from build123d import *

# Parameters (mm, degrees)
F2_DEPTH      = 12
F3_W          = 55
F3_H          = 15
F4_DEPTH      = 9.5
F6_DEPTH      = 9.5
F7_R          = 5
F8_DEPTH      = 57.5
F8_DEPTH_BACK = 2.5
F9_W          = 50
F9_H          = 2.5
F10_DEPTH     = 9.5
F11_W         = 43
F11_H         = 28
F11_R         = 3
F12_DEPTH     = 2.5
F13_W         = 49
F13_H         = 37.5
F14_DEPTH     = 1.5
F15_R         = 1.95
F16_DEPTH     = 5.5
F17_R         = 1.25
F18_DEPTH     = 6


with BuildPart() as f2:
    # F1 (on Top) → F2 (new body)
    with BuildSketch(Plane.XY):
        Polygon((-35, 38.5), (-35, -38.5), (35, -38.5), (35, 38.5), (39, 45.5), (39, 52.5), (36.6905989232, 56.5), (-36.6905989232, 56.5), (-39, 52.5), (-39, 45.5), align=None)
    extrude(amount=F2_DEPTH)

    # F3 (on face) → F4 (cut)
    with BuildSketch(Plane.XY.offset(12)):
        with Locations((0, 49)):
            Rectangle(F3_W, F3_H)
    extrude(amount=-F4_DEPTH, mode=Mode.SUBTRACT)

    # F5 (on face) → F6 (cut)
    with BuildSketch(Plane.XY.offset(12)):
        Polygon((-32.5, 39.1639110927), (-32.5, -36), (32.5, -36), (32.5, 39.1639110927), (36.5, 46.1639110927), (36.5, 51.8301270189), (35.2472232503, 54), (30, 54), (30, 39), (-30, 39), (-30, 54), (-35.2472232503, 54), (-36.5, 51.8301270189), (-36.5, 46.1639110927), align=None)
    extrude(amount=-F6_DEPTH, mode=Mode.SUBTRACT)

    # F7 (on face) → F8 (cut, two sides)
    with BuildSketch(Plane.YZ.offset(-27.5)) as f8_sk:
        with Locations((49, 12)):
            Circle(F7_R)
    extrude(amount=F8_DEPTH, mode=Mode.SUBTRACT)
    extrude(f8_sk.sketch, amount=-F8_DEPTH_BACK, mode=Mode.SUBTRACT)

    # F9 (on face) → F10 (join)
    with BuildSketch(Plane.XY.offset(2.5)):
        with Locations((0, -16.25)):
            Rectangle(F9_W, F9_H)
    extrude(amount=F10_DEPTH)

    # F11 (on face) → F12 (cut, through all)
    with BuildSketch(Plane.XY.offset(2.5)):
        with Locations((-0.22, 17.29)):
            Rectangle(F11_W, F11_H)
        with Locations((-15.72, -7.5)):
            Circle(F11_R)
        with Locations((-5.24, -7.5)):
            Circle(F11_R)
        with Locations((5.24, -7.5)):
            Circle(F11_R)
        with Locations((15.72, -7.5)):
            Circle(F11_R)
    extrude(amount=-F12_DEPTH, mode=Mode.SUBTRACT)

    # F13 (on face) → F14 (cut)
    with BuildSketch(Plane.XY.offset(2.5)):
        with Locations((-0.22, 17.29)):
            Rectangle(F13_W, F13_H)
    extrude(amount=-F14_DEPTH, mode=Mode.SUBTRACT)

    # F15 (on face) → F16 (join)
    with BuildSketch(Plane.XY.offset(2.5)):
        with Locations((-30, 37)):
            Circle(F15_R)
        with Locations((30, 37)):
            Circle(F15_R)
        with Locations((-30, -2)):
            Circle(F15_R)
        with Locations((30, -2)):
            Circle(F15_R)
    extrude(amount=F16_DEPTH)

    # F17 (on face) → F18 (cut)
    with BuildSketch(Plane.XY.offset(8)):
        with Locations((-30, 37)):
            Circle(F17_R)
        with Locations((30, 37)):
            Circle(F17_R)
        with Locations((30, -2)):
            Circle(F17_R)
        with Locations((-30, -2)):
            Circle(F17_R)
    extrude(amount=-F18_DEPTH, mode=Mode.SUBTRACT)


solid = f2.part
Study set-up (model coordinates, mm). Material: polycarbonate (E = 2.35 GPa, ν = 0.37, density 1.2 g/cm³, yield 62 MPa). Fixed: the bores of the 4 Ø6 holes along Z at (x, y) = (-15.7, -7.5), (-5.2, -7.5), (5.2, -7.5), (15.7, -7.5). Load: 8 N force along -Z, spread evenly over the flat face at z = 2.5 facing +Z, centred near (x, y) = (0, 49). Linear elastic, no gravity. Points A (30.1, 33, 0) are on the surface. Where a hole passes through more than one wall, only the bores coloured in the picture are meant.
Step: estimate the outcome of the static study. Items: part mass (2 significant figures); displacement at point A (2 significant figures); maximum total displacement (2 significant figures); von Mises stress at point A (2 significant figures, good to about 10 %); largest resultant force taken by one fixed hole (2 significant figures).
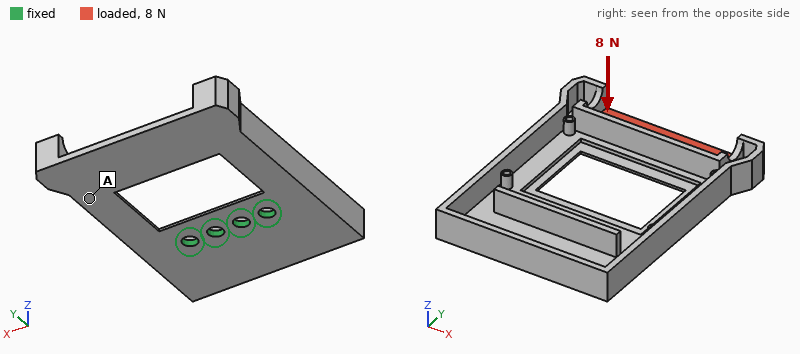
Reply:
27 g
0.82 mm
1.4 mm
1.0 MPa
10 N
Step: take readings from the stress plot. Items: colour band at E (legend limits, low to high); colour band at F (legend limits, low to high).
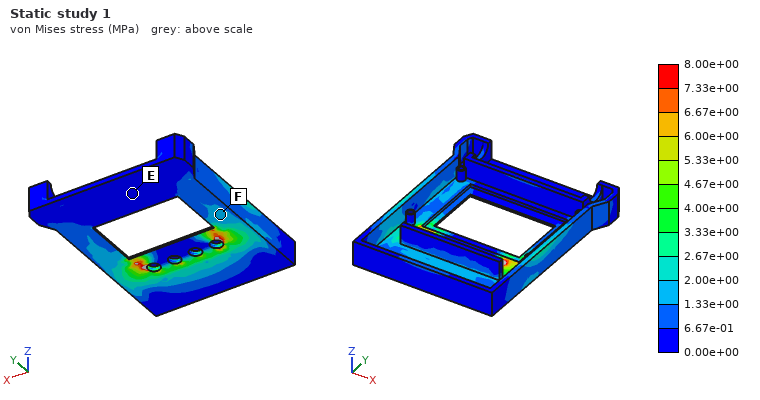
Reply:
0.00e+00 to 6.67e-01 MPa
1.33e+00 to 2.00e+00 MPa
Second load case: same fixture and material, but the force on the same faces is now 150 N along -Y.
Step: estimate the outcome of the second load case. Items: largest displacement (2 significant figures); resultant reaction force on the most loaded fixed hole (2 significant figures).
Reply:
0.57 mm
79 N
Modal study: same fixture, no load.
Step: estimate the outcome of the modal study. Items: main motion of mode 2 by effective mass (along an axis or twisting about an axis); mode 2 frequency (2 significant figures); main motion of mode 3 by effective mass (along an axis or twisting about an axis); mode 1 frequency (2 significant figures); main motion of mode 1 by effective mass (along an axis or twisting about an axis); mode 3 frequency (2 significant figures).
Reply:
twisting about Y
210 Hz
along X
140 Hz
along Z
610 Hz
